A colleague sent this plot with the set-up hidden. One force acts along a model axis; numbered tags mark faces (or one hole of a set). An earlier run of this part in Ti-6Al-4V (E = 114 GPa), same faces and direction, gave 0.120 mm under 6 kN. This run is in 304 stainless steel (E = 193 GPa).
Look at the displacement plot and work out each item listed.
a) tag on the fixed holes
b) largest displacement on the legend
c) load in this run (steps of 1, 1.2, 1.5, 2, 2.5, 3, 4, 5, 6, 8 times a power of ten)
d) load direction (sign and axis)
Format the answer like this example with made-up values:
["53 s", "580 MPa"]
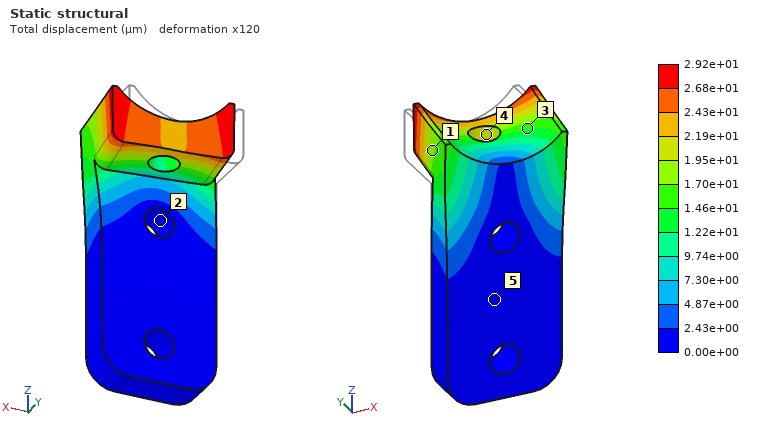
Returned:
["2", "2.92e+01 µm", "2.5 kN", "+X"]
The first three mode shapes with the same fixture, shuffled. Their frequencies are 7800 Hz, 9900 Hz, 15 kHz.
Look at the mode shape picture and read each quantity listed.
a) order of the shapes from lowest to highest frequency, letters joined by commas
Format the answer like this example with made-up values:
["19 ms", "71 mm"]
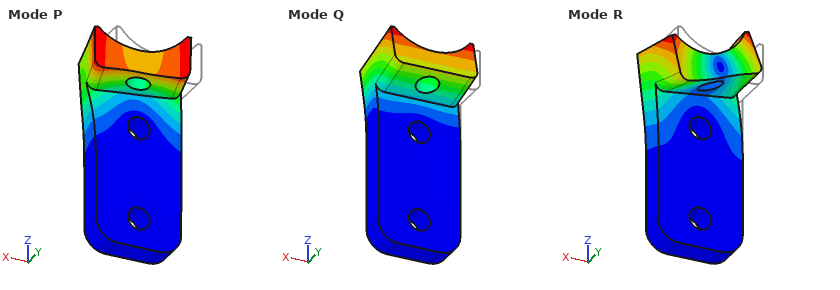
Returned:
["Q, P, R"]
